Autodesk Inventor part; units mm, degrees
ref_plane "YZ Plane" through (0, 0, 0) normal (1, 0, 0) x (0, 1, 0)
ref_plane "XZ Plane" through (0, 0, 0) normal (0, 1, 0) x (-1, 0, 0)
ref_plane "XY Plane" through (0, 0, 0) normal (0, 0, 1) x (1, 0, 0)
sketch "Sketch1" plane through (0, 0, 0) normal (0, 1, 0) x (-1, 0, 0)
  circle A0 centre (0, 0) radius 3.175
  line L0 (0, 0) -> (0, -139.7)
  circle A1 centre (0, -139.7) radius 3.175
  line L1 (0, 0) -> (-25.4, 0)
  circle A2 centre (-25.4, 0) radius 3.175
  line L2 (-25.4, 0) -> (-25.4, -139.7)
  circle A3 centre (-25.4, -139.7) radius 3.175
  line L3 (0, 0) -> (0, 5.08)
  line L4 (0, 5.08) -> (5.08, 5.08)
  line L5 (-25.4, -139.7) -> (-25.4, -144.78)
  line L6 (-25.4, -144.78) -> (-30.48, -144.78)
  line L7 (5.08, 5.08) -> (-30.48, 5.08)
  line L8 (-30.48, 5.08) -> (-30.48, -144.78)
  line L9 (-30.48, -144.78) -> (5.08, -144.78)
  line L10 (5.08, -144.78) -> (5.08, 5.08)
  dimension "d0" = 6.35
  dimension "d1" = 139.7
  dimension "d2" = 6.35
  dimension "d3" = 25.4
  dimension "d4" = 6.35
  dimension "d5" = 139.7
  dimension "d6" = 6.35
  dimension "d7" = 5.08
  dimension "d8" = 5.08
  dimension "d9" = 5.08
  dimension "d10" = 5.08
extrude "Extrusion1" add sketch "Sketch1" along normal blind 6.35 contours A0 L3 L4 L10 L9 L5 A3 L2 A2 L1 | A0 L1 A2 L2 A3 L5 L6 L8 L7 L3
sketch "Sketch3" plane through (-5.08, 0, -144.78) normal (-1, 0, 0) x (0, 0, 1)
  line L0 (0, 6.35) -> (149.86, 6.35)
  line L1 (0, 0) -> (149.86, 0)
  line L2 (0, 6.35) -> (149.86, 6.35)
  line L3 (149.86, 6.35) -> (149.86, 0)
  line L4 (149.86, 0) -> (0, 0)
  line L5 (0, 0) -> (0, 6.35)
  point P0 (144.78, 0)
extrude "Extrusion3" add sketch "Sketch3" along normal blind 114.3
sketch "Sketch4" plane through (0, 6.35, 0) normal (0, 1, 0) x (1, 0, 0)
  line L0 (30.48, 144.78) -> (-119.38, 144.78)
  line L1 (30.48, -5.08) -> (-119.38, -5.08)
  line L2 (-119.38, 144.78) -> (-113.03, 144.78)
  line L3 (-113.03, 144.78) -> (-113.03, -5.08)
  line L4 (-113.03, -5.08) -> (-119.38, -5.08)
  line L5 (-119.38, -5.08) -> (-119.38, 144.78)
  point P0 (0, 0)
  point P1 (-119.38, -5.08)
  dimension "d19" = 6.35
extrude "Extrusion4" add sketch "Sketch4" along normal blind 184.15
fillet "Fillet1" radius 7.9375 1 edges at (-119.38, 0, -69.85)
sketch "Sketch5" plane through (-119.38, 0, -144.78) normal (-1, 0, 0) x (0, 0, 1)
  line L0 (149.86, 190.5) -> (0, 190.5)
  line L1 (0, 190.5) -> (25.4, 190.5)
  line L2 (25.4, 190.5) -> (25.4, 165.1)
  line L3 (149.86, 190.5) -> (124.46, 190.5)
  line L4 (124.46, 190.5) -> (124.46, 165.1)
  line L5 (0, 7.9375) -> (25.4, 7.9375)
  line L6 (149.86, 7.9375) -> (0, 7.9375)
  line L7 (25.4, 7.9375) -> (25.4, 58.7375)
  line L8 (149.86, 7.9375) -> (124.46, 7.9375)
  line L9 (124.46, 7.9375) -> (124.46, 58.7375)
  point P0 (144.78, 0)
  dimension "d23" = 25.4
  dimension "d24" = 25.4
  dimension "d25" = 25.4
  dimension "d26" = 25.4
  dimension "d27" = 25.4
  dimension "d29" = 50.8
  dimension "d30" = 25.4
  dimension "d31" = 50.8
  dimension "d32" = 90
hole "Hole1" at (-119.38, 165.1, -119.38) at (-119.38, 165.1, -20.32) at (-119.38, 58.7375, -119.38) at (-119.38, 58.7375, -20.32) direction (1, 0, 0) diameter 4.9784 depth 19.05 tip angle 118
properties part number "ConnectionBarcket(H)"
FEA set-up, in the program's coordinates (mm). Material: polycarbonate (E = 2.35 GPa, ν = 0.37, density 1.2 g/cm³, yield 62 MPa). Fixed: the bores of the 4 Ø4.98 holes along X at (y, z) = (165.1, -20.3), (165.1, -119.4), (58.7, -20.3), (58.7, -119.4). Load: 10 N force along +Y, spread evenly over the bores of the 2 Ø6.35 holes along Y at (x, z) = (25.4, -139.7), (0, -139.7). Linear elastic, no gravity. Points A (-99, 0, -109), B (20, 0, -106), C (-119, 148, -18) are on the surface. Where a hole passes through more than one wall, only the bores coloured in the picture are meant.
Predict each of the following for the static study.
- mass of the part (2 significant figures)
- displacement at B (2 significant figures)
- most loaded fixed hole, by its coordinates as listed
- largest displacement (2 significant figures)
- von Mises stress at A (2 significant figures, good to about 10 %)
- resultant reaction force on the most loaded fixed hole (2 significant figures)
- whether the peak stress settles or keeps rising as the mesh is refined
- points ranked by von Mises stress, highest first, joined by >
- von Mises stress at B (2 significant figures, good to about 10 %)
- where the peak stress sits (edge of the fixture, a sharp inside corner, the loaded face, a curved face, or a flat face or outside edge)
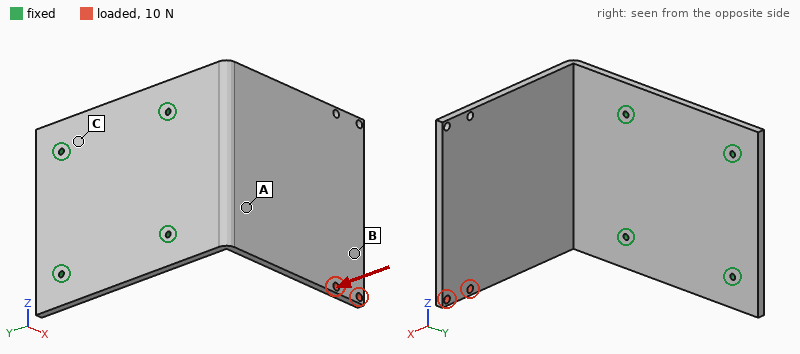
380 g
2.5 mm
(58.7, -119.4)
3.1 mm
1.2 MPa
9.5 N
keeps rising
A > B > C
0.58 MPa
edge of the fixture
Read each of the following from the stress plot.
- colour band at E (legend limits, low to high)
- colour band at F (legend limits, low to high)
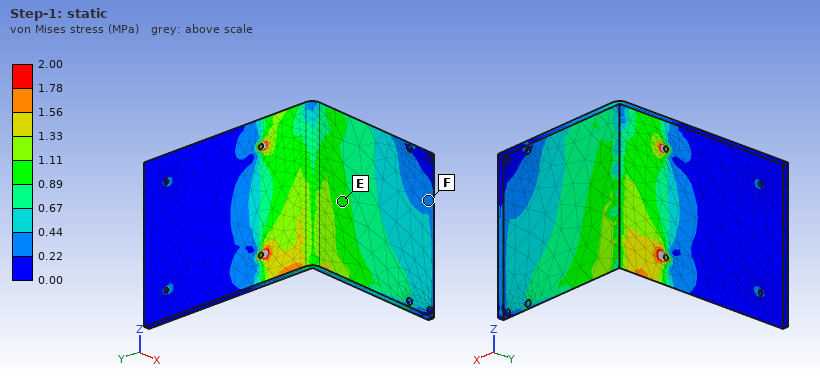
0.89 to 1.11 MPa
0.22 to 0.44 MPa
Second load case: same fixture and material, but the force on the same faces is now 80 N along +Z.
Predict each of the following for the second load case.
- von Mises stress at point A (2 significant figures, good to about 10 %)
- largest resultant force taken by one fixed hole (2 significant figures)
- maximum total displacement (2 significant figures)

2.2 MPa
120 N
3.1 mm
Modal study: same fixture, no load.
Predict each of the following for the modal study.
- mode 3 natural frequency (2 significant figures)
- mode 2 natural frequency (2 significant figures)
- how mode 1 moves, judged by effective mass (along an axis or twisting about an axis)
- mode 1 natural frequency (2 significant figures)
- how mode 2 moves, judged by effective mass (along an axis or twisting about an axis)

160 Hz
94 Hz
along Y
41 Hz
along Z
